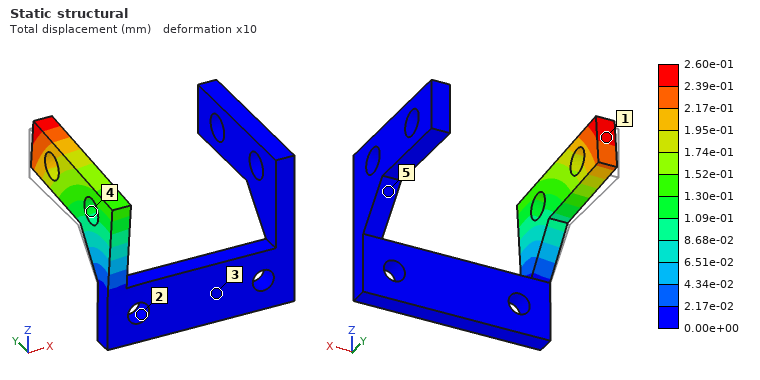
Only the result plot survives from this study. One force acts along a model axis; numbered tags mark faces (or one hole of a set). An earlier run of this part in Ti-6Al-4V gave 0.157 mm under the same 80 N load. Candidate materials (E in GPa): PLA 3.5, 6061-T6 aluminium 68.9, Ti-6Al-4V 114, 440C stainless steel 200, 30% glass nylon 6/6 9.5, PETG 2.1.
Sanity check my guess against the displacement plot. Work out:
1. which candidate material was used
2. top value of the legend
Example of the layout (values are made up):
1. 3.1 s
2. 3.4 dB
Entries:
1. 6061-T6 aluminium
2. 2.60e-01 mm
